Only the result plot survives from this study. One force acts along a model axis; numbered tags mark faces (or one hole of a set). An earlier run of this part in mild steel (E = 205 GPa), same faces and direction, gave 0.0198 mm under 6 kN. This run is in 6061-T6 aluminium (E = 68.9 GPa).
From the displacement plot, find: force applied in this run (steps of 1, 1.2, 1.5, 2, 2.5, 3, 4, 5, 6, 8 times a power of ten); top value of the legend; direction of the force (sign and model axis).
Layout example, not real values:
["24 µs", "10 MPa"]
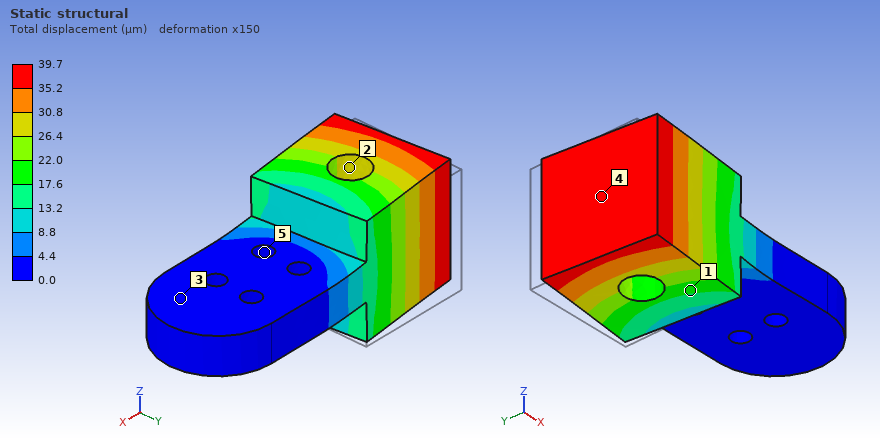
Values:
["4 kN", "39.7 µm", "-Y"]
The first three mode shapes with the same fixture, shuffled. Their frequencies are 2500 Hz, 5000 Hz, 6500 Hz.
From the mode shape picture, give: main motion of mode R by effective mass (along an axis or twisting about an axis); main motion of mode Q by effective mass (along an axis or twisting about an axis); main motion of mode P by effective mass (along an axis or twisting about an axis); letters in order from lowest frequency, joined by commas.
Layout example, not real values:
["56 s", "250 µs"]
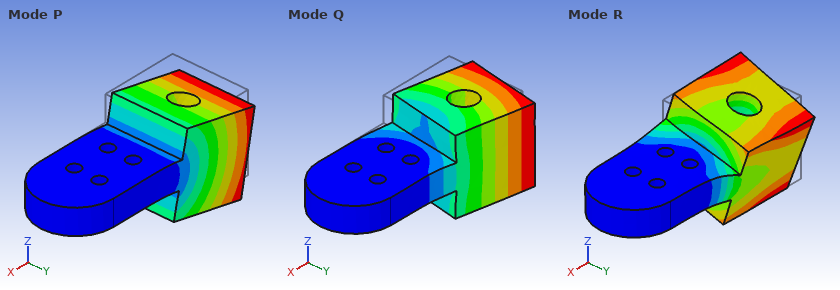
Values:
["twisting about X", "along Y", "along Z", "P, Q, R"]
